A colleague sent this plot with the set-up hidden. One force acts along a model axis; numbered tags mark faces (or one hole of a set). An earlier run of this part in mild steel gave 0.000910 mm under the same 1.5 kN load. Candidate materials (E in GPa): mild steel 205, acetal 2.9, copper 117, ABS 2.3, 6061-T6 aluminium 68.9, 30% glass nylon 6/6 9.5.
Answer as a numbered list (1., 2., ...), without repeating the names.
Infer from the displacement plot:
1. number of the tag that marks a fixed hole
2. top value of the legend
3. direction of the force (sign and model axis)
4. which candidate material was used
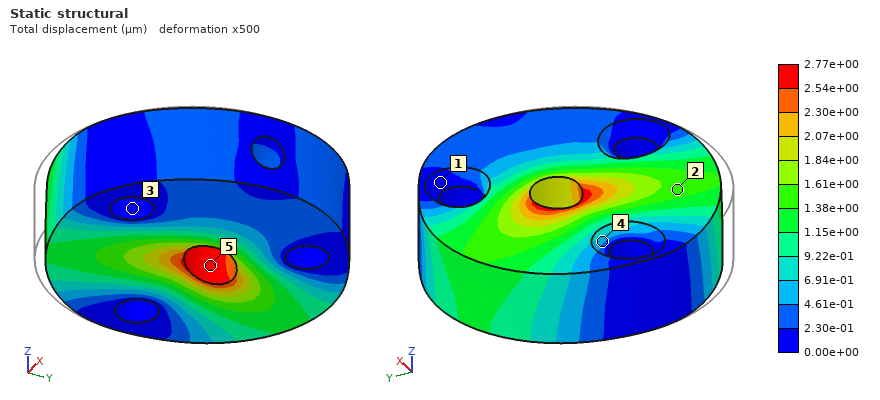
1. 3
2. 2.77e+00 µm
3. +Y
4. 6061-T6 aluminium
